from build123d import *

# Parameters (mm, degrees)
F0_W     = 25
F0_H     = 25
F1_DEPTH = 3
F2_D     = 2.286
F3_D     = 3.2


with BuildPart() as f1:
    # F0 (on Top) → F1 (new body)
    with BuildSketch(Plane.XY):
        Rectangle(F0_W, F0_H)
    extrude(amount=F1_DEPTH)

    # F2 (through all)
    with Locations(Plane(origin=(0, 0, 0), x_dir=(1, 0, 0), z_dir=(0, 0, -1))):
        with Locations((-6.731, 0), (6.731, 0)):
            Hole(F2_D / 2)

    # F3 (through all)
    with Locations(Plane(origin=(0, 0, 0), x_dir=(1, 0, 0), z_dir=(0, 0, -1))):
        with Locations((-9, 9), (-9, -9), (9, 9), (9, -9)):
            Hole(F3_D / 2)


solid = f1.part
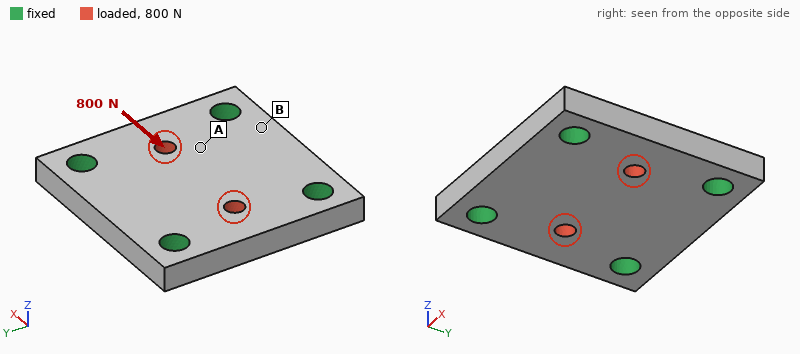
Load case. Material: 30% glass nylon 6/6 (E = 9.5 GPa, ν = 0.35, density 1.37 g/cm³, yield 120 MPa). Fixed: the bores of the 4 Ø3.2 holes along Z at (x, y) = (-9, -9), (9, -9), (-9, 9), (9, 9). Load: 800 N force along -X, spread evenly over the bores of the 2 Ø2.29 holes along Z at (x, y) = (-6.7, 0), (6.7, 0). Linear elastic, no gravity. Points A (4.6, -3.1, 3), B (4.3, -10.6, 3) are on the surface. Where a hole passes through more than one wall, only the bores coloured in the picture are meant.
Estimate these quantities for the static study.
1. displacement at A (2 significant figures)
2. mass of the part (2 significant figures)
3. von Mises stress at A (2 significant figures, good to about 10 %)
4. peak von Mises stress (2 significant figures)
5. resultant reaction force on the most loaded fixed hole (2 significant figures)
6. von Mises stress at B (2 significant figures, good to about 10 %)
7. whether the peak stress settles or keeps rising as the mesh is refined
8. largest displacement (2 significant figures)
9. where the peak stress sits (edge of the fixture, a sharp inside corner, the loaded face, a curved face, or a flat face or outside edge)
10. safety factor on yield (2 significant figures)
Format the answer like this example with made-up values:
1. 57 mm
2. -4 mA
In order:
1. 11 µm
2. 2.4 g
3. 12 MPa
4. 34 MPa
5. 210 N
6. 3.5 MPa
7. settles
8. 19 µm
9. the loaded face
10. 3.6
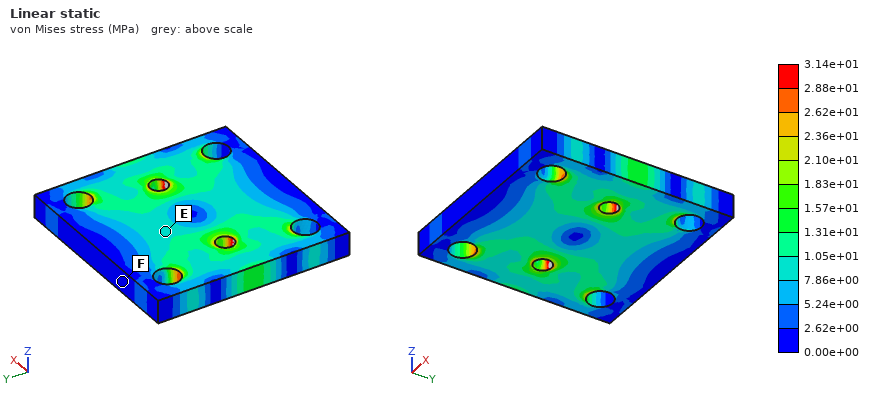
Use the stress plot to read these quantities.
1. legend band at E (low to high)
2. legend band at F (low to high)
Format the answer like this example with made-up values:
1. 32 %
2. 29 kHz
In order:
1. 7.86e+00 to 1.05e+01 MPa
2. 0.00e+00 to 2.62e+00 MPa
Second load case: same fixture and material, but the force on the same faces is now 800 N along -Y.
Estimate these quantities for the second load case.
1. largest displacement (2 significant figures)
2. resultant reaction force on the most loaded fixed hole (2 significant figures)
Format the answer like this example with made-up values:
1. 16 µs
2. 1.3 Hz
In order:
1. 11 µm
2. 210 N
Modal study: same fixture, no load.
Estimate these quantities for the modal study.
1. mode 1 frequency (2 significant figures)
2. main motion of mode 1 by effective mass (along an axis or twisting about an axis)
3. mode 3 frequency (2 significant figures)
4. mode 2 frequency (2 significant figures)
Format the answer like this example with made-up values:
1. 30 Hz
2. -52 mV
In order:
1. 18 kHz
2. along Z
3. 27 kHz
4. 27 kHz
